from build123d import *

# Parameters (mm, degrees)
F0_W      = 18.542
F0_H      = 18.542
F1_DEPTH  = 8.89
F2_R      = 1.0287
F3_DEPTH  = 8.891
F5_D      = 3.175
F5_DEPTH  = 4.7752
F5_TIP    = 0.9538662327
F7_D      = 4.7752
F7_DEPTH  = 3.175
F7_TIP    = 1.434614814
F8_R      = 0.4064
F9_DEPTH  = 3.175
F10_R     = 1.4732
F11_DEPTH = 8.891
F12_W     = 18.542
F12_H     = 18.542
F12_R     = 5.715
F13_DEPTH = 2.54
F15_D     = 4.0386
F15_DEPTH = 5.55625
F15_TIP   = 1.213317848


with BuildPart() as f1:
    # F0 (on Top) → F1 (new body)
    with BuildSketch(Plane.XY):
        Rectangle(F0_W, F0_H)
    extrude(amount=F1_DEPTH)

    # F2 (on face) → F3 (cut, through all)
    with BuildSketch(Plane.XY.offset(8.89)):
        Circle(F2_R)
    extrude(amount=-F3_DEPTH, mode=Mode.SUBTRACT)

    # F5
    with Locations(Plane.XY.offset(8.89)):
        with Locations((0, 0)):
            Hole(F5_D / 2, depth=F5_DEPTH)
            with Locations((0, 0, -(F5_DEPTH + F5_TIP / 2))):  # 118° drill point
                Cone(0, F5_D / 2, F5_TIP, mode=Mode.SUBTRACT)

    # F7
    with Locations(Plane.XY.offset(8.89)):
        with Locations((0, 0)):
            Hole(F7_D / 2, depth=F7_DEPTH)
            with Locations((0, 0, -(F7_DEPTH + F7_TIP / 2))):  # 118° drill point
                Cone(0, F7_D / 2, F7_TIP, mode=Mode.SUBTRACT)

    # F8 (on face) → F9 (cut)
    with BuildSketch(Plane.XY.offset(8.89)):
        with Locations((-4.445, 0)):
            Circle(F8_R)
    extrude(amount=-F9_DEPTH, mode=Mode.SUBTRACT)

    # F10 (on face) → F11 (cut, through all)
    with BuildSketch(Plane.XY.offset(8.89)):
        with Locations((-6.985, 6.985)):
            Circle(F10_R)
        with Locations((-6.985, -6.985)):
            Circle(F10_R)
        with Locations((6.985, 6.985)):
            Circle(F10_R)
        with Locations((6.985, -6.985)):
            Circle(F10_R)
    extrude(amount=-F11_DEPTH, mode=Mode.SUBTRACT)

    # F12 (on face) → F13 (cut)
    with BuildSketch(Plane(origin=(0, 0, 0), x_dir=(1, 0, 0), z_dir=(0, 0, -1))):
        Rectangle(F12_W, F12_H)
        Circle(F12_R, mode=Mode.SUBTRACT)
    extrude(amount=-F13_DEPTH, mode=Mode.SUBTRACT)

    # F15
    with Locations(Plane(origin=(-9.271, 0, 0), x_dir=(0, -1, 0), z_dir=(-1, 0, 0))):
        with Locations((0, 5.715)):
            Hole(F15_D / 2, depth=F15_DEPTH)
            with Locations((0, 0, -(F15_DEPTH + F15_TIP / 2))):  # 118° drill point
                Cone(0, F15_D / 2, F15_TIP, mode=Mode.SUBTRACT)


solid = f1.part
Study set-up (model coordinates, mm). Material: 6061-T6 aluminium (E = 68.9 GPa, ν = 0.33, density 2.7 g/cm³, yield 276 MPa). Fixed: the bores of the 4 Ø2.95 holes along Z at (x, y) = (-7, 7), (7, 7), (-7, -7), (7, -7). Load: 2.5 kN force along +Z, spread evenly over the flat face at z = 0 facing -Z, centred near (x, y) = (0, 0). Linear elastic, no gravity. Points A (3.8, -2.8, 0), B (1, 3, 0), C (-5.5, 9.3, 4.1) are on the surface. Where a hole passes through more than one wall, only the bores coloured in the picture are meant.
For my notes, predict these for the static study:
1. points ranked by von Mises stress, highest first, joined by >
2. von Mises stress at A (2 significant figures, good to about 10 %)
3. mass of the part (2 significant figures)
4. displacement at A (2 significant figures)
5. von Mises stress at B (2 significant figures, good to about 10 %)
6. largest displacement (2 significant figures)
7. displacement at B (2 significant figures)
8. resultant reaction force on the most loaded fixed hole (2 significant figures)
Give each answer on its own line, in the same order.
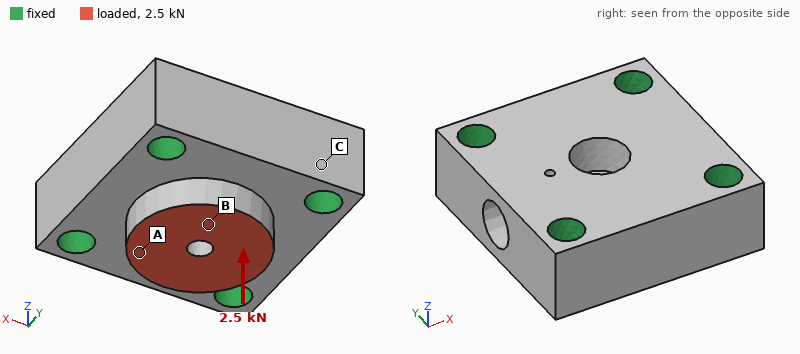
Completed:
A > B > C
23 MPa
5.7 g
4.4 µm
15 MPa
5.2 µm
4.7 µm
670 N
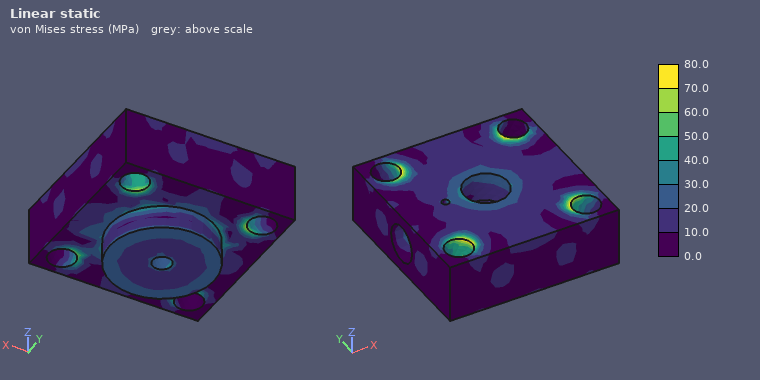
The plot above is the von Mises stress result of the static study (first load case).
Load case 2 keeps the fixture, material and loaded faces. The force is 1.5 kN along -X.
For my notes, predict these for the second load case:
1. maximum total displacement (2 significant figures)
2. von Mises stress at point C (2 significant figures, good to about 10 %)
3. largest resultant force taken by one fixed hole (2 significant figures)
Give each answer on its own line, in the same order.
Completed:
6.7 µm
4.2 MPa
520 N
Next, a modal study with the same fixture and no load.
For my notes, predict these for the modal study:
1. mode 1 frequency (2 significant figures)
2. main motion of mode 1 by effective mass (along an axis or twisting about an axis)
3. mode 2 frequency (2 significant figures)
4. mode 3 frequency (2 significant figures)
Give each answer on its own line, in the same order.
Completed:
77 kHz
along Z
92 kHz
95 kHz
